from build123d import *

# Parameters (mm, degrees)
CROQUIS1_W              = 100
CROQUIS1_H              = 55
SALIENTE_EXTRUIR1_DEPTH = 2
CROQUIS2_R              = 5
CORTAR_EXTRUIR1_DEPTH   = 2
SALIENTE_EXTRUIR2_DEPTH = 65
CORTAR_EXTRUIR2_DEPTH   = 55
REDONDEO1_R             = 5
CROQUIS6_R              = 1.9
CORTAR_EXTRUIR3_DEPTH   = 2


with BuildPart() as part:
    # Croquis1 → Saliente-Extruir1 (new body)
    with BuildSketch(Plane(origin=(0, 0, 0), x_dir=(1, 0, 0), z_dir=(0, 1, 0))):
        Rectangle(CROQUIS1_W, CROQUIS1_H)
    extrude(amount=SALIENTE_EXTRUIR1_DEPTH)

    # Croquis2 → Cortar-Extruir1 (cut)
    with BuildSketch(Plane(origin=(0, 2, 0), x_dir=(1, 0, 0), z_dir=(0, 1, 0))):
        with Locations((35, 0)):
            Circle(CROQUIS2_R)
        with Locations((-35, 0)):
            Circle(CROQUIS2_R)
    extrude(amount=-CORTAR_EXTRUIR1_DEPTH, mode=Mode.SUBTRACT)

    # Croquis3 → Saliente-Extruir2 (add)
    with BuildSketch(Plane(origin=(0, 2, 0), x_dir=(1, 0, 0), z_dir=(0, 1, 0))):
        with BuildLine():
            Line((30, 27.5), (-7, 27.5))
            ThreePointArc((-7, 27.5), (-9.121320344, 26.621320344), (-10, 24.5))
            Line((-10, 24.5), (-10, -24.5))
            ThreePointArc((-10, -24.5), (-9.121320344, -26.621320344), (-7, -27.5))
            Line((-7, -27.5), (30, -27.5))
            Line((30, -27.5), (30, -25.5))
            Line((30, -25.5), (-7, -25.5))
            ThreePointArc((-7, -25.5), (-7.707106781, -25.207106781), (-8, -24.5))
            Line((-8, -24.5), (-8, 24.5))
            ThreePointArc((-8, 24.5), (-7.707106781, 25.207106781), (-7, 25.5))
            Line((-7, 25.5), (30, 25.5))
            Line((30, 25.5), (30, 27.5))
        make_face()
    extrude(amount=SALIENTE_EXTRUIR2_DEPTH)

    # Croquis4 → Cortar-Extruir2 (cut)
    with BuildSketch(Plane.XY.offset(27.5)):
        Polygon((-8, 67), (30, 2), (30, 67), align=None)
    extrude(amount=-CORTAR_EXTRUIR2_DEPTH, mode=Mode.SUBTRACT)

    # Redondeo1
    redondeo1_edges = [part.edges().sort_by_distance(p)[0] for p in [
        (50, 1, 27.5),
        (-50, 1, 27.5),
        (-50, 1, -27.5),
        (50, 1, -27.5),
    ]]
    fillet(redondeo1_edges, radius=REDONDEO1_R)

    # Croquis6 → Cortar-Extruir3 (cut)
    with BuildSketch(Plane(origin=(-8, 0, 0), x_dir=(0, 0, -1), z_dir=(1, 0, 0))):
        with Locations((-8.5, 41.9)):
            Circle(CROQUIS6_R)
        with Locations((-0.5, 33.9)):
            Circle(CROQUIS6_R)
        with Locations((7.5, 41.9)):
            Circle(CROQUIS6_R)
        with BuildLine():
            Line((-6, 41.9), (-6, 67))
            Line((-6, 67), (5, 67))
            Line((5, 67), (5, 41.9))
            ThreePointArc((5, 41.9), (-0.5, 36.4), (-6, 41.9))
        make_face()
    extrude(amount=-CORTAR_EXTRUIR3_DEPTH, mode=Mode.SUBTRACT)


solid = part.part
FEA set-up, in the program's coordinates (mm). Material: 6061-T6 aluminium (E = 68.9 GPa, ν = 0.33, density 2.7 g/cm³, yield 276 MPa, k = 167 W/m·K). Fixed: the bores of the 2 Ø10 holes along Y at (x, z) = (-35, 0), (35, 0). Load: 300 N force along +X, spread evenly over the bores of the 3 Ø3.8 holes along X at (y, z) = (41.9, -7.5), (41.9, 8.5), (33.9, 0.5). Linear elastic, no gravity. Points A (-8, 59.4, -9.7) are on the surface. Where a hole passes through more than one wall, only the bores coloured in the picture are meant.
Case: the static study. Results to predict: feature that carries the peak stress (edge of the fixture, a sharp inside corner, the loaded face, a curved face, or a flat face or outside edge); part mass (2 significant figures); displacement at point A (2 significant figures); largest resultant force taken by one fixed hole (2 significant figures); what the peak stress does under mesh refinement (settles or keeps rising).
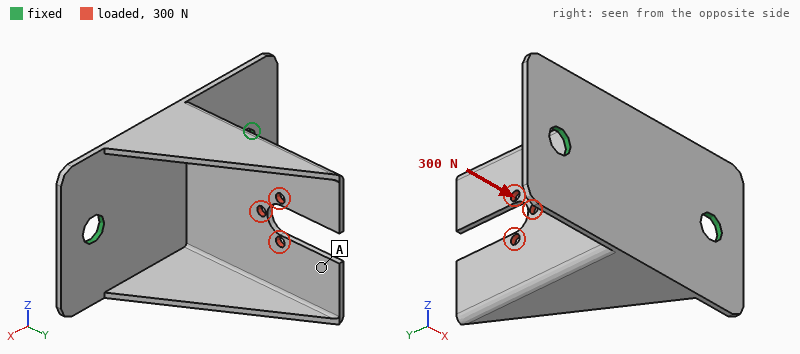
a sharp inside corner
59 g
0.80 mm
260 N
keeps rising
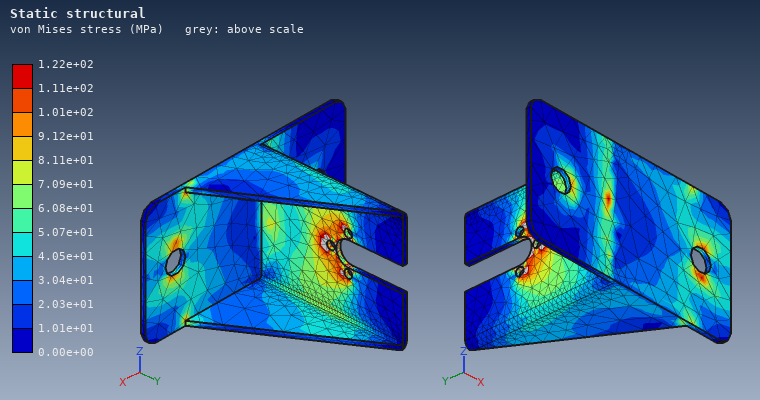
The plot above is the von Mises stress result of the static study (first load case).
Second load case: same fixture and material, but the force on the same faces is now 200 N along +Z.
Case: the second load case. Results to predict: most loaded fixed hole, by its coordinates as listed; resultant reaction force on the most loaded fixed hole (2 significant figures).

(-35, 0)
120 N
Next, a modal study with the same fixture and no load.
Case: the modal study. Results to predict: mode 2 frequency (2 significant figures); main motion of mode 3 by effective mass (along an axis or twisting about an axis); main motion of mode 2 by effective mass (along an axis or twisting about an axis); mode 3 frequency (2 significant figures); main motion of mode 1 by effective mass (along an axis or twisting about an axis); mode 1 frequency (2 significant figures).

970 Hz
along Y
along X
1300 Hz
along Z
530 Hz
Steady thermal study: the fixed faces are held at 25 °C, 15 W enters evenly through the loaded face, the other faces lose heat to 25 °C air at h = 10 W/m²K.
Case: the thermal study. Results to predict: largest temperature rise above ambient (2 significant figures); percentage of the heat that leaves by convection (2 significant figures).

36 K
19 %
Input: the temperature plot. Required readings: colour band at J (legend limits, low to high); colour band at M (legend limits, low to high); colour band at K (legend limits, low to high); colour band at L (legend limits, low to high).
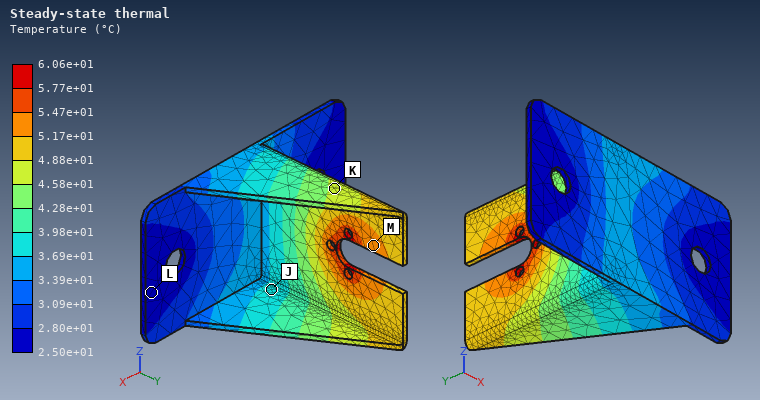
3.69e+01 to 3.98e+01 °C
5.17e+01 to 5.47e+01 °C
4.58e+01 to 4.88e+01 °C
2.50e+01 to 2.80e+01 °C
